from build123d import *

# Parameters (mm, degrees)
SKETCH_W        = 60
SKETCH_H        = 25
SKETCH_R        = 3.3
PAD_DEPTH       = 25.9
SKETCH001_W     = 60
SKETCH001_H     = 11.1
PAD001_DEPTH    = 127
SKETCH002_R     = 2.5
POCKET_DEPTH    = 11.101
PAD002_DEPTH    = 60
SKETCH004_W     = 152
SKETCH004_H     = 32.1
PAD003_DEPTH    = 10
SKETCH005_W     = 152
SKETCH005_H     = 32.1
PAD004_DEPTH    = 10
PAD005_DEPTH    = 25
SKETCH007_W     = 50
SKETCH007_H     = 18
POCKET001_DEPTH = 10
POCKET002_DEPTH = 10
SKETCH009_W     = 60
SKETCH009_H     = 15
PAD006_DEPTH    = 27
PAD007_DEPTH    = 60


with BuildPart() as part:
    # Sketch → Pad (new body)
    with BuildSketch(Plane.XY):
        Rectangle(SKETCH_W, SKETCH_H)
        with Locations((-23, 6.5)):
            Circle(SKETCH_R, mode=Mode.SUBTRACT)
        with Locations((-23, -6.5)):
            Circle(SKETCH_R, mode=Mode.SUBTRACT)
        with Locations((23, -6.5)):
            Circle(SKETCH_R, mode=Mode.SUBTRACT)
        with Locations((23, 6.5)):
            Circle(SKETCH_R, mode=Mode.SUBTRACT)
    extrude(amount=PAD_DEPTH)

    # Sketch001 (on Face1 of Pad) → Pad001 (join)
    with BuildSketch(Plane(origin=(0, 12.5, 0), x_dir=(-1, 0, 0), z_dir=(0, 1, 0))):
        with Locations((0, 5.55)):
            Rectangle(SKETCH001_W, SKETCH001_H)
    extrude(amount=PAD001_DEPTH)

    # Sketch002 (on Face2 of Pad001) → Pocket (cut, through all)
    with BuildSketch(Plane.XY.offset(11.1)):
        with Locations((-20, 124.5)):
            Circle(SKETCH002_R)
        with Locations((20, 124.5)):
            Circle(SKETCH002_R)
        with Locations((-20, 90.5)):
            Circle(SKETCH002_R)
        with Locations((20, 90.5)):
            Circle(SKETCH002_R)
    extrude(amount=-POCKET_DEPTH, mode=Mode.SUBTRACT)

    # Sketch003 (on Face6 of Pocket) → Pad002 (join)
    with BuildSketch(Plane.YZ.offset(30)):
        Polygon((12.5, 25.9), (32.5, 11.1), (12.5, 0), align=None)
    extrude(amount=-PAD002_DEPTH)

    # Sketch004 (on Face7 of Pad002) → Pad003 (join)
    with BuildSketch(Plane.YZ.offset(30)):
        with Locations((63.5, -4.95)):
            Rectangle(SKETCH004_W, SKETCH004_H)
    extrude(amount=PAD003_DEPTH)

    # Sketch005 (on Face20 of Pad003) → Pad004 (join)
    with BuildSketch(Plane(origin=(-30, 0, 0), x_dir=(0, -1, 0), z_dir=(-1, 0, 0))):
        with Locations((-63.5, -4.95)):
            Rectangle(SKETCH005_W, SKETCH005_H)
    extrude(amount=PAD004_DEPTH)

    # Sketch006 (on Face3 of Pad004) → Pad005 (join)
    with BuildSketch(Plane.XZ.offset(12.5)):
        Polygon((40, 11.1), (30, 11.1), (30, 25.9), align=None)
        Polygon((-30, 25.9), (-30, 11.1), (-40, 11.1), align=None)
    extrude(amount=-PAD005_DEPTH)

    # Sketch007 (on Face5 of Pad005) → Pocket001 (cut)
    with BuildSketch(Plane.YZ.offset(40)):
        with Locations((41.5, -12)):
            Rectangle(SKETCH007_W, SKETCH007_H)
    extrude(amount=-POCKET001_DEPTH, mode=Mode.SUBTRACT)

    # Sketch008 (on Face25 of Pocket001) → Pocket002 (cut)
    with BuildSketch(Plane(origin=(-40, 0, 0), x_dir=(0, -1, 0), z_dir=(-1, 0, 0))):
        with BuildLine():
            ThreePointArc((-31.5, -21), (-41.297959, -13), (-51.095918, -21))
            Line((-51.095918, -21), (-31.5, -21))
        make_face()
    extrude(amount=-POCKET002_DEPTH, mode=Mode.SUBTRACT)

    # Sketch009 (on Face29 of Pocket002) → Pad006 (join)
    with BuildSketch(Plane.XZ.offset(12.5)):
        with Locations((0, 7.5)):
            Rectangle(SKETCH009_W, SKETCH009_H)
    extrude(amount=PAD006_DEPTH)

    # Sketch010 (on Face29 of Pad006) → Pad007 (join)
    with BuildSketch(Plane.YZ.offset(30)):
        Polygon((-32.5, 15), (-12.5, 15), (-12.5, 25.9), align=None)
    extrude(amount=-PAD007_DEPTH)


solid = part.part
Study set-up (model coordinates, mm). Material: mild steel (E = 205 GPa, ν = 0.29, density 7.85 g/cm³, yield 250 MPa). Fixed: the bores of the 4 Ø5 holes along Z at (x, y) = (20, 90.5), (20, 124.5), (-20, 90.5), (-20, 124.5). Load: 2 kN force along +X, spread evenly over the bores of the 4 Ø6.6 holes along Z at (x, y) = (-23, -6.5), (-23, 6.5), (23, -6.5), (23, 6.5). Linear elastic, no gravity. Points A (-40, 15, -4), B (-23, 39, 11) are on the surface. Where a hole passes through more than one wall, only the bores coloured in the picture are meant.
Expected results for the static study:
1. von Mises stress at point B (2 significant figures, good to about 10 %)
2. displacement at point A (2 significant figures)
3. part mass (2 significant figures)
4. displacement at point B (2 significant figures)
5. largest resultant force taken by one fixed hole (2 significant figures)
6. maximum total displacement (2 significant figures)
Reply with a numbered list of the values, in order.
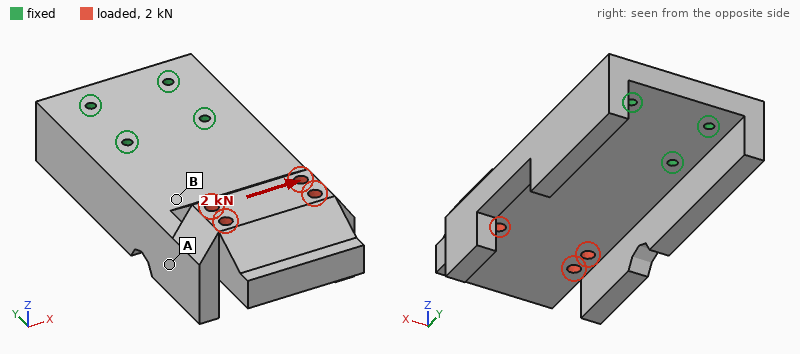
1. 7.1 MPa
2. 6.9 µm
3. 2.0 kg
4. 5.2 µm
5. 2.9 kN
6. 15 µm
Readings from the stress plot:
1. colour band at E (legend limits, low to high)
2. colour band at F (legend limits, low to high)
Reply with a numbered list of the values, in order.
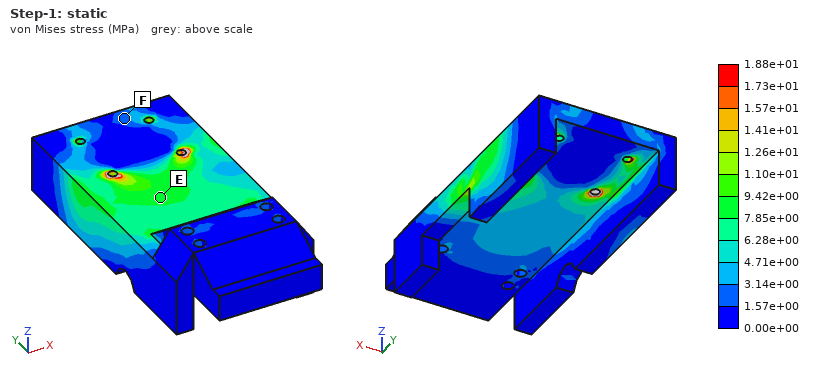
1. 7.85e+00 to 9.42e+00 MPa
2. 1.57e+00 to 3.14e+00 MPa
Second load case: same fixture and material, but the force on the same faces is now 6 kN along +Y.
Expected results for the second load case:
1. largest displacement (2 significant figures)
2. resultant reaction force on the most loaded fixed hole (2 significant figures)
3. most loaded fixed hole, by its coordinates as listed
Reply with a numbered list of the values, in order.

1. 60 µm
2. 2.8 kN
3. (-20, 90.5)
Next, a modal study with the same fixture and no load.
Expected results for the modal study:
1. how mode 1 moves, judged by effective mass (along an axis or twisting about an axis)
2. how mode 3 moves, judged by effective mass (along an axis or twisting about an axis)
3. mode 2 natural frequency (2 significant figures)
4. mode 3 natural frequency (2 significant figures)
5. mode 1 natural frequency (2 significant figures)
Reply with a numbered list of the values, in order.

1. along Z
2. along X
3. 2000 Hz
4. 2300 Hz
5. 730 Hz
